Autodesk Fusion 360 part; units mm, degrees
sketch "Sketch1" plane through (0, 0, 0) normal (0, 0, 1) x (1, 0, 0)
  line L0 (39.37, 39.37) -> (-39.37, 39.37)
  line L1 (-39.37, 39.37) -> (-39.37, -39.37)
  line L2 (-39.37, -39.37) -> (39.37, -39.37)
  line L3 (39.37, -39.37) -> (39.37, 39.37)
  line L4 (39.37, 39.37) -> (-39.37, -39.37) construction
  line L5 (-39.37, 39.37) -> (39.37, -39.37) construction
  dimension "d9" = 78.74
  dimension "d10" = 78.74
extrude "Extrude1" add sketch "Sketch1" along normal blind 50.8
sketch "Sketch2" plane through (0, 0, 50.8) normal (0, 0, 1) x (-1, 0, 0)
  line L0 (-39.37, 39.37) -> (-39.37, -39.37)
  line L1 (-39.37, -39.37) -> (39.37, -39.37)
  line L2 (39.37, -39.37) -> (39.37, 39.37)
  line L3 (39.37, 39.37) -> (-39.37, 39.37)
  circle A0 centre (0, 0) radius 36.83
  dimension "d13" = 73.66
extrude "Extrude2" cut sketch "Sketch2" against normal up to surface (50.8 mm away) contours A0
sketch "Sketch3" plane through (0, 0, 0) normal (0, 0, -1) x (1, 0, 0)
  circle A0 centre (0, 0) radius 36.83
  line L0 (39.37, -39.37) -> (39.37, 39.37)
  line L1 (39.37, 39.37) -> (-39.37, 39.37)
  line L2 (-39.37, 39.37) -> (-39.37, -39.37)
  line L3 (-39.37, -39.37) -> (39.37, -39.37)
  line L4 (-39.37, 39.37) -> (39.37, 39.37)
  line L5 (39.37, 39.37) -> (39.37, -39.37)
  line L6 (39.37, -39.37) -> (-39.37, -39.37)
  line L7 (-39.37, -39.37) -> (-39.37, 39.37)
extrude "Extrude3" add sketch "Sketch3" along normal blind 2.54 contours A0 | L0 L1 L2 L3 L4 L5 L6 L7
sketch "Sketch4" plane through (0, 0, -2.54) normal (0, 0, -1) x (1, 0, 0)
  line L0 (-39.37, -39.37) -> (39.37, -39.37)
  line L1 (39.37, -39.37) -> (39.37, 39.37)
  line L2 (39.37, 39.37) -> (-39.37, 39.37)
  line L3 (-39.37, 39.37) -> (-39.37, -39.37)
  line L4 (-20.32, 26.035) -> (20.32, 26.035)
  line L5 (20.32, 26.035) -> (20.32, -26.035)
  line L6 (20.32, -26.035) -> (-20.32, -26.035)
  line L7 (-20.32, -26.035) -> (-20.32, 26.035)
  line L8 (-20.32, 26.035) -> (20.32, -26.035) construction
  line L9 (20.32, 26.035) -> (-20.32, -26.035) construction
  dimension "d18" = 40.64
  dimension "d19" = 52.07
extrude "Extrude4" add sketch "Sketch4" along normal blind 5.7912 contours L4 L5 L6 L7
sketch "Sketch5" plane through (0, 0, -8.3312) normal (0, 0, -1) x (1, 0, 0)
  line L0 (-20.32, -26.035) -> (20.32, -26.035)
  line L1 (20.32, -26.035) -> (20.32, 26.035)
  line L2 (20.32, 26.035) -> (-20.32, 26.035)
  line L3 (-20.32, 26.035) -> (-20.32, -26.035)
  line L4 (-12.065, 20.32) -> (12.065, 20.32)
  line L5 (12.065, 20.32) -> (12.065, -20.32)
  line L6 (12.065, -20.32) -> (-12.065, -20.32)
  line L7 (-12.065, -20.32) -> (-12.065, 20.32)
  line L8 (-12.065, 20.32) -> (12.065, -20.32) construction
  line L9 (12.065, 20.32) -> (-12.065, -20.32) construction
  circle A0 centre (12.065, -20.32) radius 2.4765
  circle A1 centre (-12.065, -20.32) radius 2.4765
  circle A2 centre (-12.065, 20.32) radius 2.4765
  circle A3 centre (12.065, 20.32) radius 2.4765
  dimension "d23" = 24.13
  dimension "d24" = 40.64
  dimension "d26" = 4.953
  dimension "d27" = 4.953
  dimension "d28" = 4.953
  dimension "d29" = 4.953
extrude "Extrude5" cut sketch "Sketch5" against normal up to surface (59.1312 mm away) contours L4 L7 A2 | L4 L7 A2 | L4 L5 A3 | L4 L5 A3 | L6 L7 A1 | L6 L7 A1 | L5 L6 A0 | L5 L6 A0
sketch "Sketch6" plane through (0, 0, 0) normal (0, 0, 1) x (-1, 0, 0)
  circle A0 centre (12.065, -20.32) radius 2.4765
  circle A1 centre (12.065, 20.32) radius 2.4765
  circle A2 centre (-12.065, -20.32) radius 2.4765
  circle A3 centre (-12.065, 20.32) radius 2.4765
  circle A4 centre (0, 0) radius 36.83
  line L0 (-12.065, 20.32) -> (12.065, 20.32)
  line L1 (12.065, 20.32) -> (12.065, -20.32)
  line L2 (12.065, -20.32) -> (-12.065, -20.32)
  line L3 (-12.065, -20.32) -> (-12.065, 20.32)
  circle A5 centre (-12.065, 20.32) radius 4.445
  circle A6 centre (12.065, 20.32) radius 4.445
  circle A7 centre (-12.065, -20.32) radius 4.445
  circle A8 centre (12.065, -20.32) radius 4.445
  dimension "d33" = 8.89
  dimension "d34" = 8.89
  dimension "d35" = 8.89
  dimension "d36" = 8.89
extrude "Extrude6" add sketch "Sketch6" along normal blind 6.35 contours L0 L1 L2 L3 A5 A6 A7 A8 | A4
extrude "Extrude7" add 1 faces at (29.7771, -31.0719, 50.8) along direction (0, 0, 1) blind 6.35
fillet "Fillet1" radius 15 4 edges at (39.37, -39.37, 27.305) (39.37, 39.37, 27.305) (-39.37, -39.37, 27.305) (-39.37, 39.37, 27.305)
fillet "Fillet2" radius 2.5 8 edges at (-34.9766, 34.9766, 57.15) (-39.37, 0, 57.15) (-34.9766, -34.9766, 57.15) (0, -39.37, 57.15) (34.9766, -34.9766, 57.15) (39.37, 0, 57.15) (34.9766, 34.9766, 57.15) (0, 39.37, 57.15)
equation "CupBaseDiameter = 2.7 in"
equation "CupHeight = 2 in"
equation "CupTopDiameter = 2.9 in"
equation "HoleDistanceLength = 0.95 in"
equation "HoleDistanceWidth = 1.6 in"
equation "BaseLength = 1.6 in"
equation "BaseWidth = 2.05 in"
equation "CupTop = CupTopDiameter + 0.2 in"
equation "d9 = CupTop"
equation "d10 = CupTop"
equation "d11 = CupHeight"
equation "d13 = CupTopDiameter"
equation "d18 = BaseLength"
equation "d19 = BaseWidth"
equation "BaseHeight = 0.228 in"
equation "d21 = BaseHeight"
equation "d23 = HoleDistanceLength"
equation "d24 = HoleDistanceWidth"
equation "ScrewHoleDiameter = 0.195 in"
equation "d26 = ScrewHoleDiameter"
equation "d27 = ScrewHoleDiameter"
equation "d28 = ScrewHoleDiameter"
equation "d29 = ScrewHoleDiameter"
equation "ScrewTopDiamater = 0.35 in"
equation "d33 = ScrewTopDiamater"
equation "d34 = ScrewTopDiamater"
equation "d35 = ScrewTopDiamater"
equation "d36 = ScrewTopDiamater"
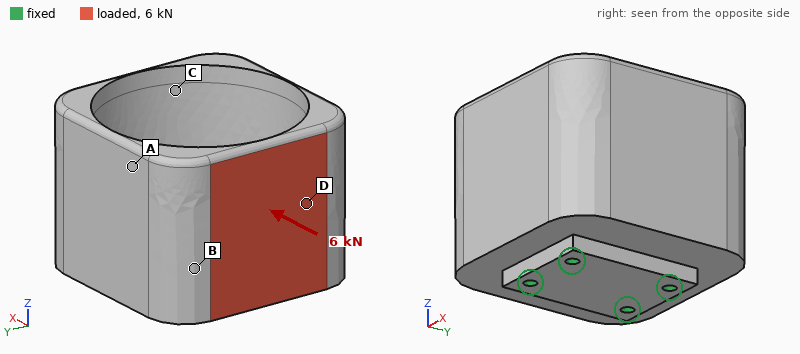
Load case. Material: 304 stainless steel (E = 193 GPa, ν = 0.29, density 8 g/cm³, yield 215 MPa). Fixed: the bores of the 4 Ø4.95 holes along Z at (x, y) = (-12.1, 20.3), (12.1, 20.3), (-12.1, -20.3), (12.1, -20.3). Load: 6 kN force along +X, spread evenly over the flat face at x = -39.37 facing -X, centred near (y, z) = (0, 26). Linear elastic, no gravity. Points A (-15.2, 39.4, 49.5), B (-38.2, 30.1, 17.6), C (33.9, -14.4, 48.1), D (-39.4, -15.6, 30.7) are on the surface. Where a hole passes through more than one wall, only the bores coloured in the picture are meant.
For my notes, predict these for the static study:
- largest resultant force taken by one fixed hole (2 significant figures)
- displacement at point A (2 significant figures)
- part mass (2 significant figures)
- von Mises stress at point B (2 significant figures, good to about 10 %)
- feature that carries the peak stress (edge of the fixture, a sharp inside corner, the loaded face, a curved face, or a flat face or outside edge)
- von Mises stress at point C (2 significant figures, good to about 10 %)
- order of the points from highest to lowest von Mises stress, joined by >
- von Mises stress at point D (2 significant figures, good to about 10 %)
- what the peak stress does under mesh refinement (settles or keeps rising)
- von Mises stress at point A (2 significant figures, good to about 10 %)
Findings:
3.4 kN
30 µm
1.2 kg
33 MPa
edge of the fixture
5.9 MPa
B > D > A > C
24 MPa
keeps rising
12 MPa
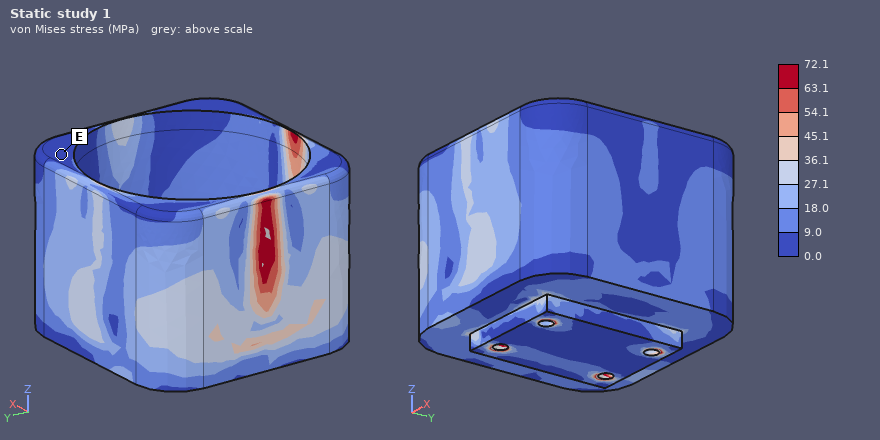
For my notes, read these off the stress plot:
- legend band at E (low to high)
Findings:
0.0 to 9.0 MPa
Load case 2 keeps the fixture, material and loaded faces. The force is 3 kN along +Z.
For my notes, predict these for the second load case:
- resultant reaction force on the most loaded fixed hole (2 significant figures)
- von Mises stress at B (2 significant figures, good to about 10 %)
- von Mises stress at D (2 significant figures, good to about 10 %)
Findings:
2.8 kN
6.6 MPa
8.1 MPa
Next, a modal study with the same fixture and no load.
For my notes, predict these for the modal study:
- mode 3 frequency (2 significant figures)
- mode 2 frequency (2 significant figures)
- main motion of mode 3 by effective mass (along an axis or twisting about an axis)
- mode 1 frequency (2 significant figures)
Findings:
3500 Hz
2800 Hz
along Y
2700 Hz
